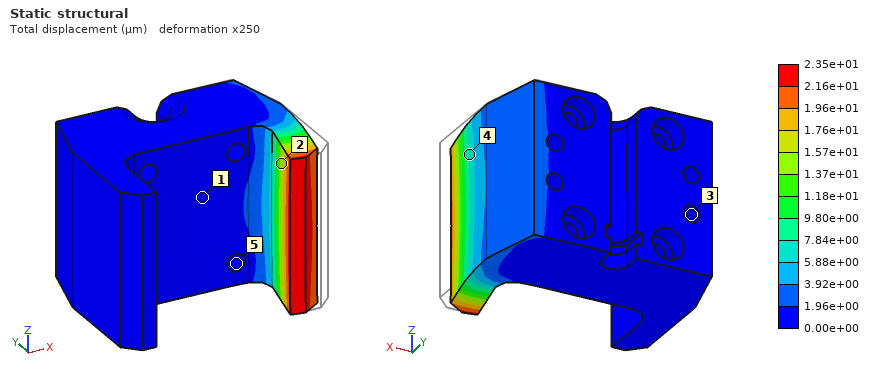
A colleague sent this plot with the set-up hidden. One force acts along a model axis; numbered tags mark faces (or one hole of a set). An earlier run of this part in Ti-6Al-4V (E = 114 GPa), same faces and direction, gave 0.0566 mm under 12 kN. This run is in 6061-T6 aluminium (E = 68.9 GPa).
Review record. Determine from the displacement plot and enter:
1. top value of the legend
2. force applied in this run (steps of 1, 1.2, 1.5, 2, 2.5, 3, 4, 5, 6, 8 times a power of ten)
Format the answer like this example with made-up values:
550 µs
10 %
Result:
2.35e+01 µm
3 kN
